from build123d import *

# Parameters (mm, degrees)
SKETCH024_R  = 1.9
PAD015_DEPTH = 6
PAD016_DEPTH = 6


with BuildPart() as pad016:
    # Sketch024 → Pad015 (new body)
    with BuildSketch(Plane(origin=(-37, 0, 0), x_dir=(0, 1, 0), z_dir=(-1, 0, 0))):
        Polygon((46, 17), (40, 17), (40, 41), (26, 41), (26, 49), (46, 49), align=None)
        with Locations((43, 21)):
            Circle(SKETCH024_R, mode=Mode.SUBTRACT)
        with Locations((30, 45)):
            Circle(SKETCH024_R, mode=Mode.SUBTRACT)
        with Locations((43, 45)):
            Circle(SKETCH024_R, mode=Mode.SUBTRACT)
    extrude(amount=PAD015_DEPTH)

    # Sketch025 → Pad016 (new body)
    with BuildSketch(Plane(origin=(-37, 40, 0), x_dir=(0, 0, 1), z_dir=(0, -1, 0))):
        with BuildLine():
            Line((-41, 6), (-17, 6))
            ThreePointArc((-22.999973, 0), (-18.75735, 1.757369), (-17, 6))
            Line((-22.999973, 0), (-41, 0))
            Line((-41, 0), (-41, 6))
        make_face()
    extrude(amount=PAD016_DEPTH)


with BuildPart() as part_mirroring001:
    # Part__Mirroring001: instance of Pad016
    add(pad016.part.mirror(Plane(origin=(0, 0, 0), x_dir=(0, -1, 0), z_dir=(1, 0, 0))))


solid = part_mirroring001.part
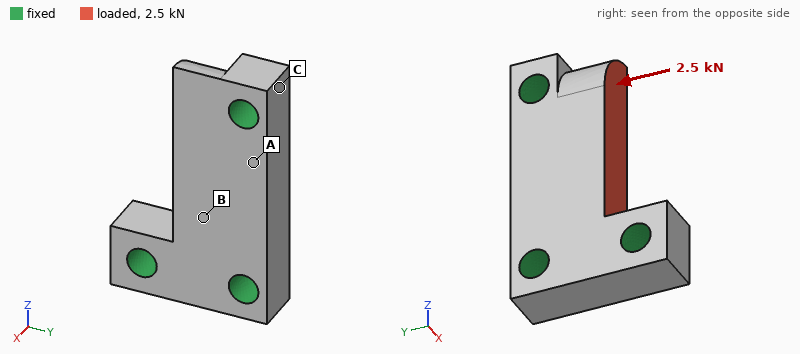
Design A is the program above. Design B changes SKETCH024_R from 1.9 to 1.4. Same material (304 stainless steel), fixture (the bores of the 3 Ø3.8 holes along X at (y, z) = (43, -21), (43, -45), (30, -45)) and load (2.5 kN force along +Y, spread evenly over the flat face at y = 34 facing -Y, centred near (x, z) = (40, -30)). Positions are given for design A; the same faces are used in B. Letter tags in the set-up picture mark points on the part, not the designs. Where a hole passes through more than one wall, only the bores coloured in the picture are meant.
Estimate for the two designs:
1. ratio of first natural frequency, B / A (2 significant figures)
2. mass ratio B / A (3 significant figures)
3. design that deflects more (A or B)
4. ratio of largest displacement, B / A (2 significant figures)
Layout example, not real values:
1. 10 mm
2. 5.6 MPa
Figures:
1. 0.91
2. 1.04
3. B
4. 1.1
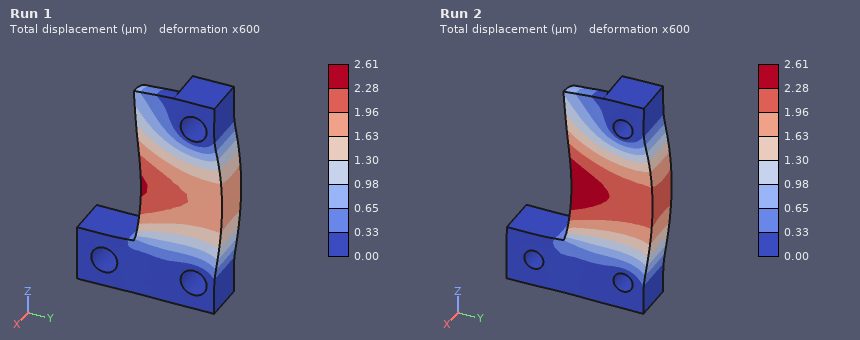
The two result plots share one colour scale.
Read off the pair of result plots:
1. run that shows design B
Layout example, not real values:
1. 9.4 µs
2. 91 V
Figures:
1. Run 2
